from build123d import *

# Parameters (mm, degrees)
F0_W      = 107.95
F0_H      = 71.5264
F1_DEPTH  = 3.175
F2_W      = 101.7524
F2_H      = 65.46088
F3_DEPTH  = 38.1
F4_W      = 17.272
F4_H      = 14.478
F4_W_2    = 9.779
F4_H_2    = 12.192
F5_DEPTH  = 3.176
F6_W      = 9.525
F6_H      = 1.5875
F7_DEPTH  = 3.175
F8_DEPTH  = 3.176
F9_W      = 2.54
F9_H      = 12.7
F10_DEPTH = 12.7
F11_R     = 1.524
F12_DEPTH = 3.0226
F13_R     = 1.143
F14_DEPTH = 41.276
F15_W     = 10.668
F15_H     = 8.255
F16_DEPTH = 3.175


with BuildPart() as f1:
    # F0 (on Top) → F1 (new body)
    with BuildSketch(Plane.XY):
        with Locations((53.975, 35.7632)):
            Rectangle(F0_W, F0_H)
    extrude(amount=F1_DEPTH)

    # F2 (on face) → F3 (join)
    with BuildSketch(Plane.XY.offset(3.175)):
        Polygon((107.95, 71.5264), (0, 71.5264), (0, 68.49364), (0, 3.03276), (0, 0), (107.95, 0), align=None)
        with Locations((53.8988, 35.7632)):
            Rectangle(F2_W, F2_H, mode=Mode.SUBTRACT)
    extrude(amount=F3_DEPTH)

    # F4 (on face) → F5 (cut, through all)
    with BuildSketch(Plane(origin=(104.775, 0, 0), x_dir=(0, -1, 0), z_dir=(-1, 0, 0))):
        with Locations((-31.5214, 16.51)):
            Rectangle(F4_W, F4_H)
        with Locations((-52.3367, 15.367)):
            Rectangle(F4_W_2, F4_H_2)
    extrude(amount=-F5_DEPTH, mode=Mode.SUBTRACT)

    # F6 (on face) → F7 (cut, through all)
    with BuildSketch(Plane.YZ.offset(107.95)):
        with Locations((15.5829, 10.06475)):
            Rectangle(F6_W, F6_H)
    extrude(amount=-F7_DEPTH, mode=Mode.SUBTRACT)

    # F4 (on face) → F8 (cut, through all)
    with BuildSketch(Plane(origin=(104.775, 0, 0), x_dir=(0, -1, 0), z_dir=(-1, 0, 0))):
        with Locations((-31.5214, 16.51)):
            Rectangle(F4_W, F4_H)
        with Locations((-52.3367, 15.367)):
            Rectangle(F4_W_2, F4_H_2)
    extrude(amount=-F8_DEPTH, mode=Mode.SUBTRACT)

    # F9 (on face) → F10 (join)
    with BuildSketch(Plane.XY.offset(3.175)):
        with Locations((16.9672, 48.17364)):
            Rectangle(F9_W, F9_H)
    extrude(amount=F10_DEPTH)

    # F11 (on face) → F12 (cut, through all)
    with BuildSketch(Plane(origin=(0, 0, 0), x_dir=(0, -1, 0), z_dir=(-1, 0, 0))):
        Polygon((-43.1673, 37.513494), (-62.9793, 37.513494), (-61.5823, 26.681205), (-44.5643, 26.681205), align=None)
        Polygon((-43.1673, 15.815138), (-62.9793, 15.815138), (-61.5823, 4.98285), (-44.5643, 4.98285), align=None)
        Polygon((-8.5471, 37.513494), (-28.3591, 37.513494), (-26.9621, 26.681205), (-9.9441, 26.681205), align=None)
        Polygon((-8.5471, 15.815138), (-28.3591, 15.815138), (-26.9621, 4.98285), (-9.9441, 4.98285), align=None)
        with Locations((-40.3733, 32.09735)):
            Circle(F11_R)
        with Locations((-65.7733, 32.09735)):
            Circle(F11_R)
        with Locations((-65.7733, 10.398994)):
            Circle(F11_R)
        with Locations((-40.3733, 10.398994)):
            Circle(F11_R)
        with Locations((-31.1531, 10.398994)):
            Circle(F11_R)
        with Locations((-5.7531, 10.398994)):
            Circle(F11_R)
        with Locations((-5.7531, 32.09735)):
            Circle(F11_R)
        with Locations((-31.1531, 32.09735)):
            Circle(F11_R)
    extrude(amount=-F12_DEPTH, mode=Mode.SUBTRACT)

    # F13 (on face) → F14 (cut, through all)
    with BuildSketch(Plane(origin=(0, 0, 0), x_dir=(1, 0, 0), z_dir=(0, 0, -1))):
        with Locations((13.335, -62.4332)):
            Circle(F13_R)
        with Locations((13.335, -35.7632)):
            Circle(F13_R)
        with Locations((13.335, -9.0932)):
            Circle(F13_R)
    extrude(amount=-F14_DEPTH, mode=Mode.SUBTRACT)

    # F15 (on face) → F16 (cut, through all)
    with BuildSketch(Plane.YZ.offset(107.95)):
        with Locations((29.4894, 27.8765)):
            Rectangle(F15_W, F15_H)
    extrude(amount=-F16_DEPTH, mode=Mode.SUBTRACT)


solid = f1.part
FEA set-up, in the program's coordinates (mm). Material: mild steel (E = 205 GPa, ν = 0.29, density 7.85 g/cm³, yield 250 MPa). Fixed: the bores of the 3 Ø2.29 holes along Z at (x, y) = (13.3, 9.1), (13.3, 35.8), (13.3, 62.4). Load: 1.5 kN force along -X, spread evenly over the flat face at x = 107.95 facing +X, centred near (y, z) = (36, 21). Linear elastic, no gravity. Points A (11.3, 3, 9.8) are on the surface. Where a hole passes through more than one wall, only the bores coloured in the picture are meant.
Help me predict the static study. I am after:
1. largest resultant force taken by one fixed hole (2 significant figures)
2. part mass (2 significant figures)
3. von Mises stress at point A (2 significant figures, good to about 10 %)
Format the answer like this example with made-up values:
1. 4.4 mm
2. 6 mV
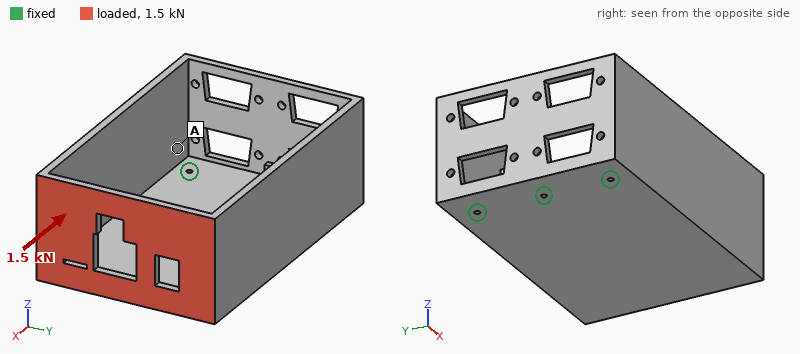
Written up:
1. 690 N
2. 480 g
3. 23 MPa
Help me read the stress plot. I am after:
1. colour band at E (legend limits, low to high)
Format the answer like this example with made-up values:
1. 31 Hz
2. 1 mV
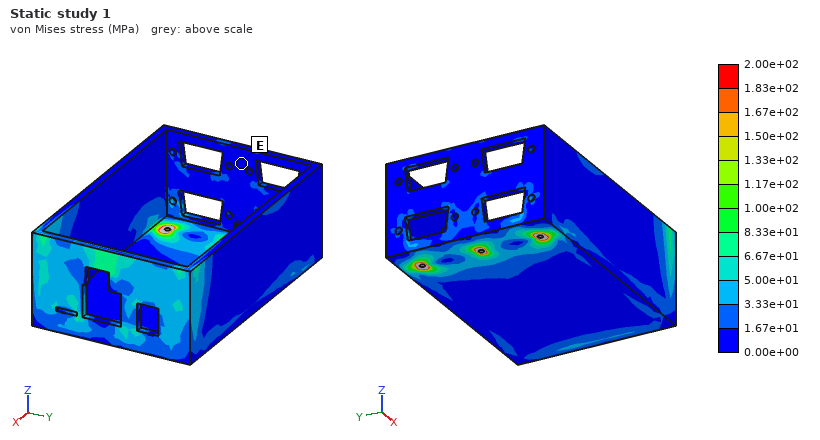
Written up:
1. 0.00e+00 to 1.67e+01 MPa
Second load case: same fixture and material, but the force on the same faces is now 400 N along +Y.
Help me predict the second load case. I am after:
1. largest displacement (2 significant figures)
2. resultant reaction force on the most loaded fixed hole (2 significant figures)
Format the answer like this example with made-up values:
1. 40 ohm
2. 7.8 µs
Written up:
1. 0.15 mm
2. 730 N
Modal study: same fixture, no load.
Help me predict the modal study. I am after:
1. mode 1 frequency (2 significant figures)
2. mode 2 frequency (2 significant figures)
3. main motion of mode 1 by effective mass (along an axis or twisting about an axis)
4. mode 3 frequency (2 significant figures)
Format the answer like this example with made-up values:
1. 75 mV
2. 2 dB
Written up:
1. 330 Hz
2. 610 Hz
3. along Z
4. 1900 Hz
